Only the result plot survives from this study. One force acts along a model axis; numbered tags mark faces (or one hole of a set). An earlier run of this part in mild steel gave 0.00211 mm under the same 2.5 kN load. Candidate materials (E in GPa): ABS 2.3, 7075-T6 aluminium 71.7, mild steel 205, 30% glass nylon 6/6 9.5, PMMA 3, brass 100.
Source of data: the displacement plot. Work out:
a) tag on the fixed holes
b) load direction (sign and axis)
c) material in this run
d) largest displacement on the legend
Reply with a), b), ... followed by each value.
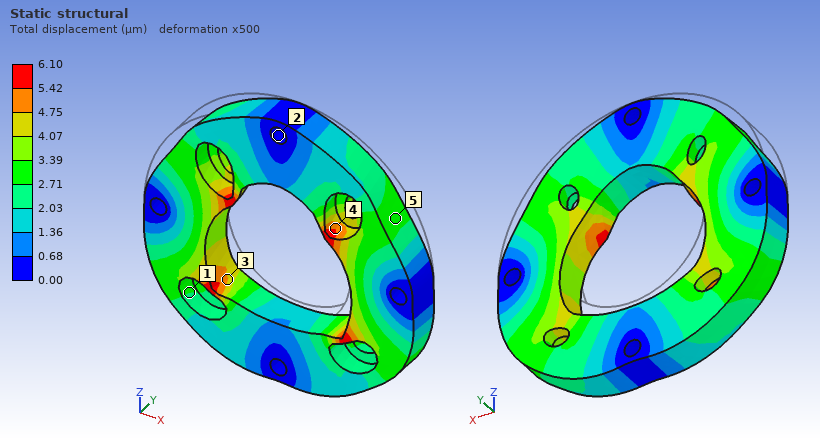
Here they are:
a) 2
b) -Z
c) 7075-T6 aluminium
d) 6.10 µm
